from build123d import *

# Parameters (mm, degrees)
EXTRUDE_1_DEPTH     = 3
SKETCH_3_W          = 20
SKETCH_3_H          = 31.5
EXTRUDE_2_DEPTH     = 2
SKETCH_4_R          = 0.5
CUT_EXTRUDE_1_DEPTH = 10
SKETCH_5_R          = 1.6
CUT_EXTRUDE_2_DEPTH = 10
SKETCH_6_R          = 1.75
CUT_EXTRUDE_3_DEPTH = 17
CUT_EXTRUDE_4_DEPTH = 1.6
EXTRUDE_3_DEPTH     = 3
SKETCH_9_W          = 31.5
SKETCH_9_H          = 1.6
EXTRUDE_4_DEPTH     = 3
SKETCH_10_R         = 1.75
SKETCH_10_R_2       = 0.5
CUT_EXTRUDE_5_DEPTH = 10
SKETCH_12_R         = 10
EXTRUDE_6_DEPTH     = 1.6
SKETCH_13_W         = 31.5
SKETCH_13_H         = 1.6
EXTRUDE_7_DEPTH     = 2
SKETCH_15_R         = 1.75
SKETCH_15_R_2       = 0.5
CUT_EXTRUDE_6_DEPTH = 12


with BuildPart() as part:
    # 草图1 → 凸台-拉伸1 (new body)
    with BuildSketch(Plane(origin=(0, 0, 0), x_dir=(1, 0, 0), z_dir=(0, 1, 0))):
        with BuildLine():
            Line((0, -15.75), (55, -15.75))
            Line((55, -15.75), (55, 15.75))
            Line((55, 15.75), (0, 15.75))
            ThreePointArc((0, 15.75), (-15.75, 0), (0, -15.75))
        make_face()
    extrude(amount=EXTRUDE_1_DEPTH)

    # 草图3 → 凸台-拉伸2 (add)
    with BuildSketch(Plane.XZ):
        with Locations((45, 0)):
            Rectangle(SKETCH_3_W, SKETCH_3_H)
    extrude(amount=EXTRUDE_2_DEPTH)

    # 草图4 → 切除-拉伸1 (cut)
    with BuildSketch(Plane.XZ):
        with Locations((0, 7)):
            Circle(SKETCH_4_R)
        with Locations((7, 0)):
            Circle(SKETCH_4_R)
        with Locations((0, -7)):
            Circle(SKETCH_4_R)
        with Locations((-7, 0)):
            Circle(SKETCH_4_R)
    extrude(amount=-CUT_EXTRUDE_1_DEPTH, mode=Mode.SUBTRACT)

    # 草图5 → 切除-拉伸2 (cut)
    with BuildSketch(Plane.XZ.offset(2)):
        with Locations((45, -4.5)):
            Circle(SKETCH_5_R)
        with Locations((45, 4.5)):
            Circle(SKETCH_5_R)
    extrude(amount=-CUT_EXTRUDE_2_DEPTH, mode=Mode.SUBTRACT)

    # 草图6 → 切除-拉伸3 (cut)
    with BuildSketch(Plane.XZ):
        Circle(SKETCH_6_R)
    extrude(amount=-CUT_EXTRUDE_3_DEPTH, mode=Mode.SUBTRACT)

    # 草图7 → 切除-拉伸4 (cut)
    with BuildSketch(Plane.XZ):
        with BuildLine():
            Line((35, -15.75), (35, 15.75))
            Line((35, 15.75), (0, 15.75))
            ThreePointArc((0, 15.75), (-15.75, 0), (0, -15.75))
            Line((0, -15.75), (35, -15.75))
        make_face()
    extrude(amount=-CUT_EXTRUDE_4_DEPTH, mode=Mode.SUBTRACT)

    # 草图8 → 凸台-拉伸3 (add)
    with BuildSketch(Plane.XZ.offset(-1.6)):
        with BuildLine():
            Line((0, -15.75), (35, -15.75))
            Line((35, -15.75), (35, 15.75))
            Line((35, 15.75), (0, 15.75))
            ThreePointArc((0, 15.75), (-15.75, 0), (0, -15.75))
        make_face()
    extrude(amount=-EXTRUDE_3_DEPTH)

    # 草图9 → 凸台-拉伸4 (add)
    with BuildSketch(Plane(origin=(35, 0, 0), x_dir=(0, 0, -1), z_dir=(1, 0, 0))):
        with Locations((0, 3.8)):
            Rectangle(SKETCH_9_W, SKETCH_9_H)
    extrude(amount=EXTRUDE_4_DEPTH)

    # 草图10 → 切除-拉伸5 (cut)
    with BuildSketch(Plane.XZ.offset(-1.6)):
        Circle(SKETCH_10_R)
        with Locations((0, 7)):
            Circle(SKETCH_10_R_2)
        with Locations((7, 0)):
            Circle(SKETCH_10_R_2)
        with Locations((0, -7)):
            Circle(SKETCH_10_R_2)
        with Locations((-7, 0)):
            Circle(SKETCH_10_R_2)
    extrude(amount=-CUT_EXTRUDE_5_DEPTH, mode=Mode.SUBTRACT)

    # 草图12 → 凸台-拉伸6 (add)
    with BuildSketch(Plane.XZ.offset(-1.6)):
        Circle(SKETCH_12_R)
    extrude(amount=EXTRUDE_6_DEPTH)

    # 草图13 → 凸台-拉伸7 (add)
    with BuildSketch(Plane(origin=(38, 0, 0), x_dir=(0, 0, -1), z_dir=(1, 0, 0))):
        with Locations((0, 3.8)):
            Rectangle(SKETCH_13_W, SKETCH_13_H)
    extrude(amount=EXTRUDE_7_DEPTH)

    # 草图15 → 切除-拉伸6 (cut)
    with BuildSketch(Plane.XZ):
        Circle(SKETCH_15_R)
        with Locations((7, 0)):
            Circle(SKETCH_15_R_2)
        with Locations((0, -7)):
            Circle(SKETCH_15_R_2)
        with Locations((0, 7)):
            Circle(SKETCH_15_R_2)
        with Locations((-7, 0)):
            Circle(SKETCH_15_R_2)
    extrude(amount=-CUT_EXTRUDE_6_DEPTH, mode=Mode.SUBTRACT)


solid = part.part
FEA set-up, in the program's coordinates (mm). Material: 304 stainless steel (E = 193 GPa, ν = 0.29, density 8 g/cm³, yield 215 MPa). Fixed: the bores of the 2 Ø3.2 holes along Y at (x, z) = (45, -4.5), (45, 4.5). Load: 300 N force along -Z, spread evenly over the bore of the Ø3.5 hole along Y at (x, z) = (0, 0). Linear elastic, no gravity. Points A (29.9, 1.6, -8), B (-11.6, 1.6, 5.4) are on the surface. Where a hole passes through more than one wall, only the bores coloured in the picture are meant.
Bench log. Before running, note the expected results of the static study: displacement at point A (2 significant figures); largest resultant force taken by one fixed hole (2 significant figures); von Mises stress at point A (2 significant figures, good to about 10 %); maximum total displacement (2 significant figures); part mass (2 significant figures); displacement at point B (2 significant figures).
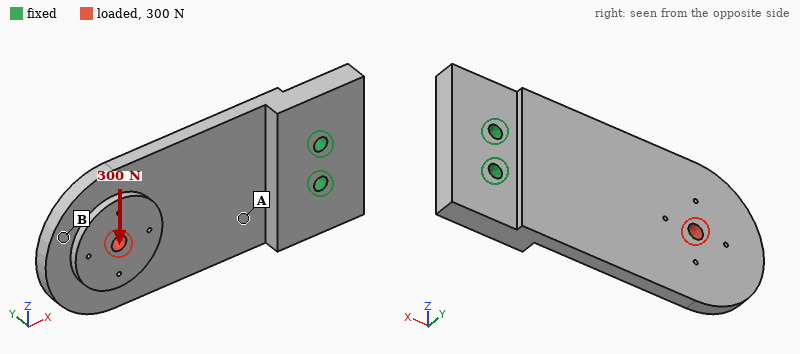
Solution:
4.3 µm
1.2 kN
16 MPa
20 µm
66 g
19 µm
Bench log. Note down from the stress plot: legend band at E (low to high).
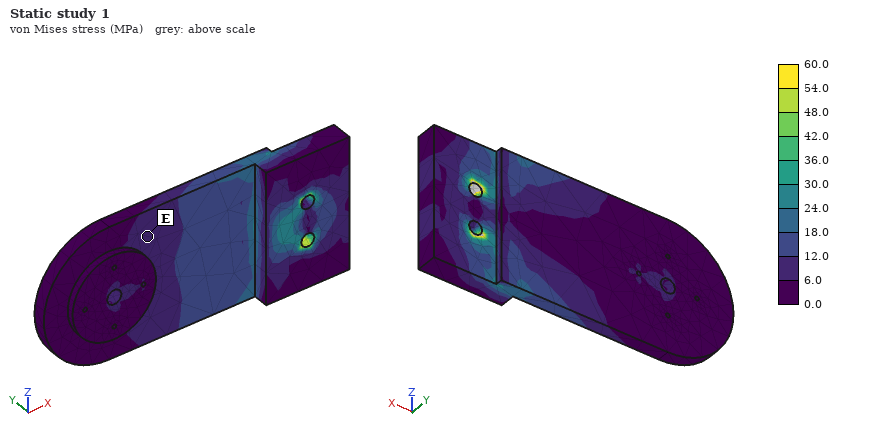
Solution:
6.0 to 12.0 MPa
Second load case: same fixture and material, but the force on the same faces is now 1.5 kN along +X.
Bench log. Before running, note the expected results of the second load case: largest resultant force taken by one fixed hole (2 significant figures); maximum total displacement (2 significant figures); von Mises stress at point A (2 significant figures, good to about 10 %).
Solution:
750 N
74 µm
39 MPa
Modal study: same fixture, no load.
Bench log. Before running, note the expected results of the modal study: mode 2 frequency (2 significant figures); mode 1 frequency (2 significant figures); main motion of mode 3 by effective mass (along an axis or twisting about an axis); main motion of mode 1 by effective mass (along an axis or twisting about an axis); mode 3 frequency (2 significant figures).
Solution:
3400 Hz
860 Hz
along Z
along Y
4600 Hz
